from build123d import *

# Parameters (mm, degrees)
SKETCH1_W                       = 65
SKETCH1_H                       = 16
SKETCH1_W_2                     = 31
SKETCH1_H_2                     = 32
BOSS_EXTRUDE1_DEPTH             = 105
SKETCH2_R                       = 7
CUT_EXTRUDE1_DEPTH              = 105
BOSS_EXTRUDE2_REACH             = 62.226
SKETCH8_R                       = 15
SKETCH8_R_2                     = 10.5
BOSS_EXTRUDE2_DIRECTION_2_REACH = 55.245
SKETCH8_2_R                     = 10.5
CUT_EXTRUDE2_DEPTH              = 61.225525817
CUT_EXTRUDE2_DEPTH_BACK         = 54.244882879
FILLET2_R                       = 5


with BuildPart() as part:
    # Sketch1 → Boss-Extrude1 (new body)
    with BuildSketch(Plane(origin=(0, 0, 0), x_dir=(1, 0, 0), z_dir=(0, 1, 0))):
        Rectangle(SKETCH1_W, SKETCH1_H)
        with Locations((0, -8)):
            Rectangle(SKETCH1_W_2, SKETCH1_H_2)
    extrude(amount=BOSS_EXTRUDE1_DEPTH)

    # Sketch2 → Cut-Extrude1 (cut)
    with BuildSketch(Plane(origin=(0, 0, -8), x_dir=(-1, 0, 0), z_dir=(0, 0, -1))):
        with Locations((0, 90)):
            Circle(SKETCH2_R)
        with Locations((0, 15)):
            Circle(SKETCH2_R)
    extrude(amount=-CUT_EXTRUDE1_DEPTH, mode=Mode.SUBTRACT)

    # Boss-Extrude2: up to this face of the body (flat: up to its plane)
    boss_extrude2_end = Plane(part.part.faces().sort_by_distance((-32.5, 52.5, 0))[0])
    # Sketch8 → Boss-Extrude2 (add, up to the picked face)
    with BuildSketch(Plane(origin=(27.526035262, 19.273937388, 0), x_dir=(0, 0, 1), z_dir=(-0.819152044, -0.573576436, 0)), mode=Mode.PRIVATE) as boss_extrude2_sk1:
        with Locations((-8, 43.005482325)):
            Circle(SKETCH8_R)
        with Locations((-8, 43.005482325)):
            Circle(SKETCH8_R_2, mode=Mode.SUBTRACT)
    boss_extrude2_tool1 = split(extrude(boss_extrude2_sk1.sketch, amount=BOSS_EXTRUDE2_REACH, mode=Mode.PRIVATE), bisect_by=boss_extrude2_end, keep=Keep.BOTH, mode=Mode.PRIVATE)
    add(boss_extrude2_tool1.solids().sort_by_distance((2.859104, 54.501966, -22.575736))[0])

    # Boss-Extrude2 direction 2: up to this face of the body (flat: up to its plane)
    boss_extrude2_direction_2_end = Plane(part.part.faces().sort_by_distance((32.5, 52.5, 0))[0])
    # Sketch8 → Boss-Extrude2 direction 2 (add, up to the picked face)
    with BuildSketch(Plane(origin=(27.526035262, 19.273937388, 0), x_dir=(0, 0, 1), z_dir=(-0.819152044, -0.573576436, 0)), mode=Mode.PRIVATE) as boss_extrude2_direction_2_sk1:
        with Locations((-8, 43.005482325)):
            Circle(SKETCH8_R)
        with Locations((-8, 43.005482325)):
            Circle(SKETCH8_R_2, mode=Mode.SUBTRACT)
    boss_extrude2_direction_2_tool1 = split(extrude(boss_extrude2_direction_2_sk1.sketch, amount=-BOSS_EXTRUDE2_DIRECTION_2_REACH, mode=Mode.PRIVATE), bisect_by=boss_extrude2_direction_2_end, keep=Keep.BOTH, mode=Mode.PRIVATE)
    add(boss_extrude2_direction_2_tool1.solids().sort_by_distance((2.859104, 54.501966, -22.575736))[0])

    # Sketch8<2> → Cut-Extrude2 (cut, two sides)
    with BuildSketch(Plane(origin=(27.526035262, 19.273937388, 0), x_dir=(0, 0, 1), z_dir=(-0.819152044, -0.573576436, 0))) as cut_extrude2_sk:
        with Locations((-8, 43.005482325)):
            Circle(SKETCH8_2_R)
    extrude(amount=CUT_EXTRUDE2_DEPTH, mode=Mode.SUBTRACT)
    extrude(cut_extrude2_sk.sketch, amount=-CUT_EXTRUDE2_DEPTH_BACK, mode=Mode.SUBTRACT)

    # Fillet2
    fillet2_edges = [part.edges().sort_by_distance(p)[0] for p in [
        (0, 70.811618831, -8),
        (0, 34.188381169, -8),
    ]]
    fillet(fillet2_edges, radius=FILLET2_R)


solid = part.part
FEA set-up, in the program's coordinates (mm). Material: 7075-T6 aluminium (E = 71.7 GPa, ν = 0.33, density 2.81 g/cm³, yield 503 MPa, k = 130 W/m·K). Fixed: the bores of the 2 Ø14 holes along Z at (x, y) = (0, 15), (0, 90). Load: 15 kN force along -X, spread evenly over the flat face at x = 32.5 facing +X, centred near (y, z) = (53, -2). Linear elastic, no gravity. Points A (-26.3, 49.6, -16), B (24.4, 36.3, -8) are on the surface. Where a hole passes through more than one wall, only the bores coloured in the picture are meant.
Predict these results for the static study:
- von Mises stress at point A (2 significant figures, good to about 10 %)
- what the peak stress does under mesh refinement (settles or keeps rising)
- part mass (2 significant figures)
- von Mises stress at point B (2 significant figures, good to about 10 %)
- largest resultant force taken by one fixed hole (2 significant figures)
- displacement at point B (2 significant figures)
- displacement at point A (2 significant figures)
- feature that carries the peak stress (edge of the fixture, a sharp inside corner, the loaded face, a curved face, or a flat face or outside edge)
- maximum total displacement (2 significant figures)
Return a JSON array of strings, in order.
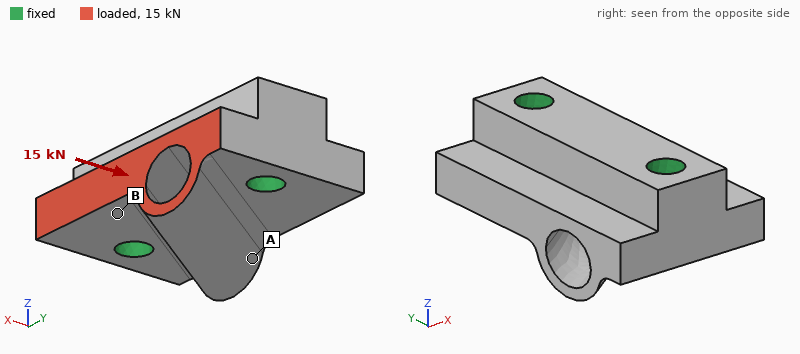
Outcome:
["4.2 MPa", "keeps rising", "430 g", "10 MPa", "7.6 kN", "9.1 µm", "7.8 µm", "edge of the fixture", "24 µm"]
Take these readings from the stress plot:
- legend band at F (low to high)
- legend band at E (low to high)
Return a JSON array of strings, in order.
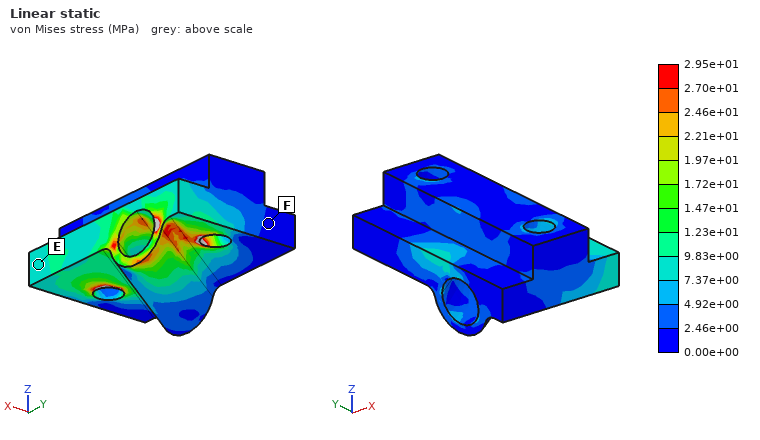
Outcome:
["0.00e+00 to 2.46e+00 MPa", "7.37e+00 to 9.83e+00 MPa"]
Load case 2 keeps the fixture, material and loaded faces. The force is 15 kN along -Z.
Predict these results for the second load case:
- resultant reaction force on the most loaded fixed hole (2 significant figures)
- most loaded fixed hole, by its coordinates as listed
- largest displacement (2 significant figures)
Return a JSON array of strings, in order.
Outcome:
["8.2 kN", "(0, 15)", "63 µm"]
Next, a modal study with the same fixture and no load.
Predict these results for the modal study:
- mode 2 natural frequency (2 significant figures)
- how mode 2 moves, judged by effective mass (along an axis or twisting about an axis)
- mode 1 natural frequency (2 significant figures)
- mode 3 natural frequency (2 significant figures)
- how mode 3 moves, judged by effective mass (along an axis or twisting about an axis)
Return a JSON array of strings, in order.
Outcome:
["14 kHz", "along Z", "11 kHz", "15 kHz", "along X"]
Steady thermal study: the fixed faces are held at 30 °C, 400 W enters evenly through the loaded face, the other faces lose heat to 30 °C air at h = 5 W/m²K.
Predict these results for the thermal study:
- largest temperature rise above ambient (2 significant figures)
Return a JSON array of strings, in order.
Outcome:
["72 K"]
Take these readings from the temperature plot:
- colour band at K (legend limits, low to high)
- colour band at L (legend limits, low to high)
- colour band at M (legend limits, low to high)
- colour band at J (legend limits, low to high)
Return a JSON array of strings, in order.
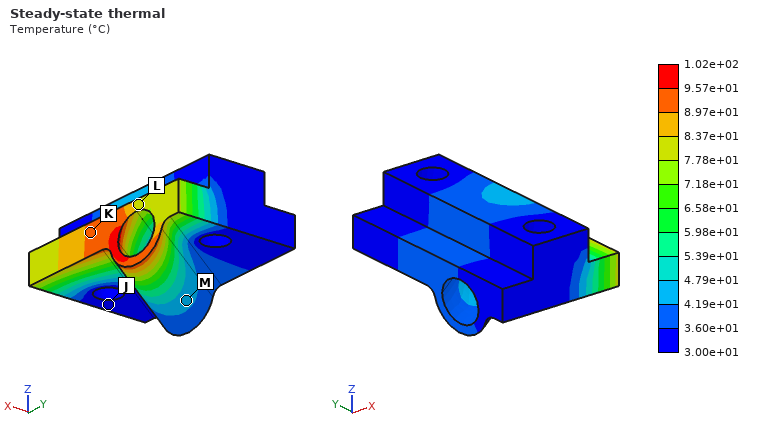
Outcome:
["8.97e+01 to 9.57e+01 °C", "7.78e+01 to 8.37e+01 °C", "4.19e+01 to 4.79e+01 °C", "3.00e+01 to 3.60e+01 °C"]
